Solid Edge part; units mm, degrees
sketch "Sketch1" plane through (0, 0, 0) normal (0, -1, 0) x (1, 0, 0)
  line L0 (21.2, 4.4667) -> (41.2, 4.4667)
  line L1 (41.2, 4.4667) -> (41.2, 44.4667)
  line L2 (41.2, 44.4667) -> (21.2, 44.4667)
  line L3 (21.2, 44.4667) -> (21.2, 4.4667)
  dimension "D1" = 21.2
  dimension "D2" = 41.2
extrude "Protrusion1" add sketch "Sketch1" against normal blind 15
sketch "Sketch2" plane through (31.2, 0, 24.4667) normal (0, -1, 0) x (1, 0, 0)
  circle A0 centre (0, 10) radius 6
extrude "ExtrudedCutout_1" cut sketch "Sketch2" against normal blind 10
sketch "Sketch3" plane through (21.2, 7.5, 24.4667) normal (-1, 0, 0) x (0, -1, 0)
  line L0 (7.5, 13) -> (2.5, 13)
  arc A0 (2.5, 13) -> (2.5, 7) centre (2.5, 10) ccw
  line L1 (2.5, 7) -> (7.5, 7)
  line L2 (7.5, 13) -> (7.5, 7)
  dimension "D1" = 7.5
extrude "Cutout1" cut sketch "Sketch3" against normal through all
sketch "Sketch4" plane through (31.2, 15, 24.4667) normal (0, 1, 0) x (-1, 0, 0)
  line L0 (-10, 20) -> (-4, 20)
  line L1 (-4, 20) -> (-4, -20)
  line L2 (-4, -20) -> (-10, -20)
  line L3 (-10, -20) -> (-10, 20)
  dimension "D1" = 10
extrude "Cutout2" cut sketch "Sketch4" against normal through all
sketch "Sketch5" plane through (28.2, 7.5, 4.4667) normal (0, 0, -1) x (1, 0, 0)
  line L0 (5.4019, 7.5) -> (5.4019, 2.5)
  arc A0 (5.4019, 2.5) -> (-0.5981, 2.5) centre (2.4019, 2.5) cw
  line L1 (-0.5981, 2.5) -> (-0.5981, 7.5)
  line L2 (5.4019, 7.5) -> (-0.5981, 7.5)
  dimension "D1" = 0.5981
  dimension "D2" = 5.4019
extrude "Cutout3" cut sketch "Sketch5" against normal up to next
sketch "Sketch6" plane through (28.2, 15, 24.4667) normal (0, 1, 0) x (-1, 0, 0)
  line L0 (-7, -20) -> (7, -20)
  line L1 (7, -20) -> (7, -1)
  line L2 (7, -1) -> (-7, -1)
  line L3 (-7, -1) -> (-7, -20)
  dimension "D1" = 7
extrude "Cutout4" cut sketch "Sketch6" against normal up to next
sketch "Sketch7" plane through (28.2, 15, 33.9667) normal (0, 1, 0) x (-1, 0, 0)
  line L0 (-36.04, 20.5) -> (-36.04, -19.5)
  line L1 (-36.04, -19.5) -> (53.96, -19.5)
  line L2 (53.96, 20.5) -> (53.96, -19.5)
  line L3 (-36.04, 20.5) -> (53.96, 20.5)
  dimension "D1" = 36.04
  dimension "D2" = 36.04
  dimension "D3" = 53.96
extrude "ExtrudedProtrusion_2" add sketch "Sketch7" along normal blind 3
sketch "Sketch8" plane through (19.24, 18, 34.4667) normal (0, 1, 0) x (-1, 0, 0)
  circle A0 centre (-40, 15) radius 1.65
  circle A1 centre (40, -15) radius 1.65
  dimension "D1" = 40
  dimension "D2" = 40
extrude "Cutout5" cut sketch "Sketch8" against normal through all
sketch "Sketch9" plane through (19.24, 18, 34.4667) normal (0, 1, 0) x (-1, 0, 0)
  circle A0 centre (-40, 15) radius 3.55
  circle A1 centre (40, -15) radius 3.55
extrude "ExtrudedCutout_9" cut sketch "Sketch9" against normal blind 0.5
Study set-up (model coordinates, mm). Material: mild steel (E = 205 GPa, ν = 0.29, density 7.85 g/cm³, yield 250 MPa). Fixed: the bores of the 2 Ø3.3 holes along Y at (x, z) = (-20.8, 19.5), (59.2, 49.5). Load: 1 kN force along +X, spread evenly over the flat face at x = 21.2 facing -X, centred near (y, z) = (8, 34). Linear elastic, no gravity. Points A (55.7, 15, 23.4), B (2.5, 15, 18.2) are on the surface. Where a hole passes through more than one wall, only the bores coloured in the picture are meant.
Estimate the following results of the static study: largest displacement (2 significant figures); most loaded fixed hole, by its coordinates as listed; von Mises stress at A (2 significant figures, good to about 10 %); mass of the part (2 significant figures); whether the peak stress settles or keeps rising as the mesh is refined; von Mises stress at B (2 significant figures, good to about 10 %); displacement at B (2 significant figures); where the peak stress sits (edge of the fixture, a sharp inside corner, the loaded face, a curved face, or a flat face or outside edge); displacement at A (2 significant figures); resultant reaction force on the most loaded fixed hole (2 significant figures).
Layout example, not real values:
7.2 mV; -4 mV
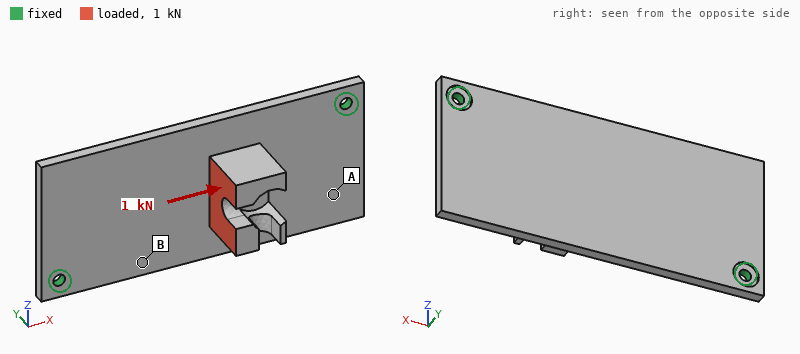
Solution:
85 µm; (59.2, 49.5); 12 MPa; 110 g; keeps rising; 37 MPa; 14 µm; edge of the fixture; 50 µm; 580 N
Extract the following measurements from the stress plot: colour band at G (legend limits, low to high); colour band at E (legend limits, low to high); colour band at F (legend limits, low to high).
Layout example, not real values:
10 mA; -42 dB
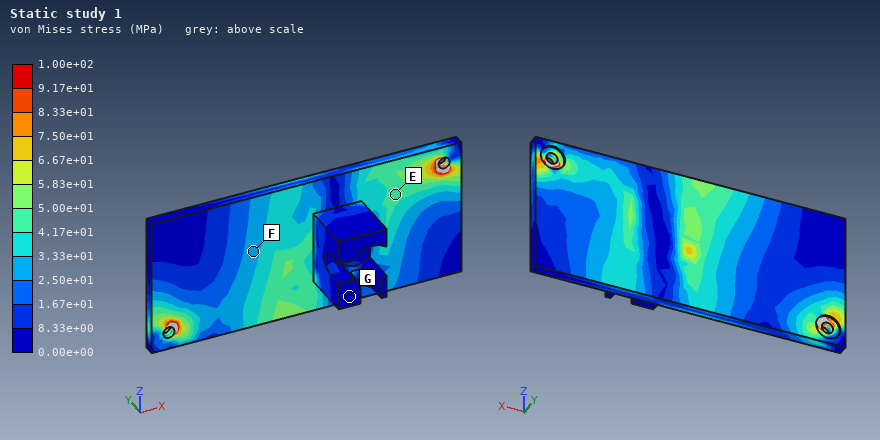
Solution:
0.00e+00 to 8.33e+00 MPa; 4.17e+01 to 5.00e+01 MPa; 2.50e+01 to 3.33e+01 MPa
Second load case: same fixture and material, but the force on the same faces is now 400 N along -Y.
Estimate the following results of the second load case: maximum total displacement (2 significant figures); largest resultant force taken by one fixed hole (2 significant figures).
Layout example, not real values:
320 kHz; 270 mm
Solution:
0.10 mm; 210 N
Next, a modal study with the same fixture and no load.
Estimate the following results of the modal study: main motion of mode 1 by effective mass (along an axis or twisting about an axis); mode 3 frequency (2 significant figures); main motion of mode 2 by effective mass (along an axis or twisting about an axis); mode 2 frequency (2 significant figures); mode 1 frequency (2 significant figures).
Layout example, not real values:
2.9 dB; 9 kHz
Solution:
along Y; 3300 Hz; along Y; 1400 Hz; 1300 Hz
